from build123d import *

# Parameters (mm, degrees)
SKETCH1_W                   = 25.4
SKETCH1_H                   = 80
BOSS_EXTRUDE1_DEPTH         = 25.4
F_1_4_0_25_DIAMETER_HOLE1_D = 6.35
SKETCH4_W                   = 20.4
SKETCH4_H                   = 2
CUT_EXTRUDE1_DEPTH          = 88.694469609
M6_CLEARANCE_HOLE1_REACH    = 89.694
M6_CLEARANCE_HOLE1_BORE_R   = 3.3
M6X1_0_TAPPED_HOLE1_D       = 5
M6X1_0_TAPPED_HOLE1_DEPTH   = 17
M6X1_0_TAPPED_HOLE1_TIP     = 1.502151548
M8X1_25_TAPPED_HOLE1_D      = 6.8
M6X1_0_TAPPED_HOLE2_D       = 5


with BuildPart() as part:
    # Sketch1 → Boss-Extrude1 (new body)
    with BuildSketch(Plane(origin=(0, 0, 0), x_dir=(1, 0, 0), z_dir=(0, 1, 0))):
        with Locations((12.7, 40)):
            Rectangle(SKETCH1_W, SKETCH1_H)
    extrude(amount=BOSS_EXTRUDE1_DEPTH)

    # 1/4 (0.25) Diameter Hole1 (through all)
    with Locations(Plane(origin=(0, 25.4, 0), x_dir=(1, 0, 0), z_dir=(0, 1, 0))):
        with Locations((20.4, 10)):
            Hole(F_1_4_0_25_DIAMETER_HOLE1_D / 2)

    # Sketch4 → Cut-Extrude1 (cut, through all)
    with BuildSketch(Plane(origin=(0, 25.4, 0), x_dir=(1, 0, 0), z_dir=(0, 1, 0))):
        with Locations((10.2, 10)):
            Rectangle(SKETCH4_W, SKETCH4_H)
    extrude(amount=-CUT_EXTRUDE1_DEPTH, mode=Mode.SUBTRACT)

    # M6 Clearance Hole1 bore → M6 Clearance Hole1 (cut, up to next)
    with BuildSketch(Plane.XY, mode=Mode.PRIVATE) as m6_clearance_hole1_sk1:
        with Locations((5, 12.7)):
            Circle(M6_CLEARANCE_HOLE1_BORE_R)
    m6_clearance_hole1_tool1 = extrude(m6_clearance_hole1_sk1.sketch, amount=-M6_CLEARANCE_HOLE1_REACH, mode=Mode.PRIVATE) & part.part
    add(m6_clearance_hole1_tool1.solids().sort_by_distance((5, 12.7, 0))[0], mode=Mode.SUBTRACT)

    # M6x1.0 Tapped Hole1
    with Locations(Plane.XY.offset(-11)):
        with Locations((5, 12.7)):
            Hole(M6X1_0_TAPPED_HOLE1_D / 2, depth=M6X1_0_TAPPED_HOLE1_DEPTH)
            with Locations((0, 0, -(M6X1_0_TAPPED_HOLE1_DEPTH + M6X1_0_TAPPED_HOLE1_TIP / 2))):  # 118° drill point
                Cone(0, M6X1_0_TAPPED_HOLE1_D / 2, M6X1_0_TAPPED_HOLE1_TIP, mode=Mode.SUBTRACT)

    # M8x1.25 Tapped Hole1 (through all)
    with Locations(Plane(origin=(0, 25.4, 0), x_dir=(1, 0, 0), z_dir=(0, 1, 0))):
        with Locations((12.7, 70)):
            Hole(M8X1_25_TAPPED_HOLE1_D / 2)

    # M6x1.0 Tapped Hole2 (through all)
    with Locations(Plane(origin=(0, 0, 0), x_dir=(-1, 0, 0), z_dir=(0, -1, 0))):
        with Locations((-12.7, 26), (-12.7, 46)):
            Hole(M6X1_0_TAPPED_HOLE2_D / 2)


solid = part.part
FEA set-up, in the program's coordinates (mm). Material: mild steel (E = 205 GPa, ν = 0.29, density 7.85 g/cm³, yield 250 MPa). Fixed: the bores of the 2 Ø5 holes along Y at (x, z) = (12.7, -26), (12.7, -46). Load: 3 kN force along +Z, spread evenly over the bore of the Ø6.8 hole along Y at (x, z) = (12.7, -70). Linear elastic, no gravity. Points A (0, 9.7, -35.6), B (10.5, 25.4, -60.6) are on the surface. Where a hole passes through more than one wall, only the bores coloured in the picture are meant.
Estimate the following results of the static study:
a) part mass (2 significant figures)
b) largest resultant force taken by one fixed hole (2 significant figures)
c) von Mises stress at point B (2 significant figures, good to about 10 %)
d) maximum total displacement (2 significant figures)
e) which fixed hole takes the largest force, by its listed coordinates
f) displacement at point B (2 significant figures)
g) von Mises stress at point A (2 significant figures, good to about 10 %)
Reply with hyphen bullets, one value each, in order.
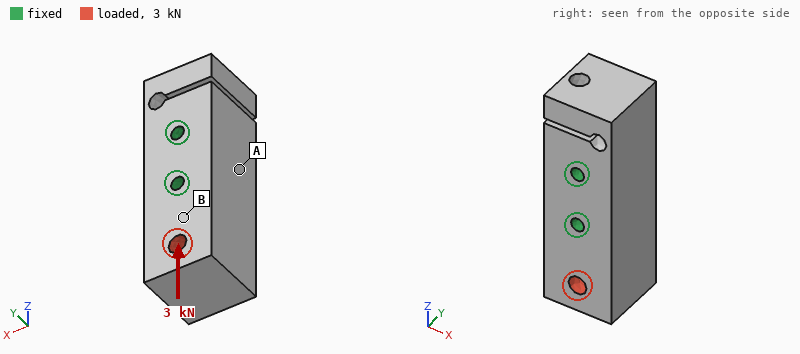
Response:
- 370 g
- 2.4 kN
- 6.5 MPa
- 0.97 µm
- (12.7, -46)
- 0.44 µm
- 1.4 MPa
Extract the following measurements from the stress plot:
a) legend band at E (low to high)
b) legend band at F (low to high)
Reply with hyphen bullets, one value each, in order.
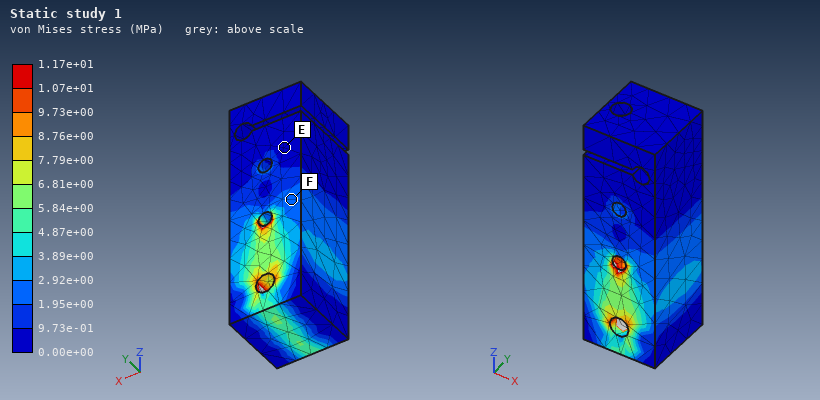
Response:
- 0.00e+00 to 9.73e-01 MPa
- 1.95e+00 to 2.92e+00 MPa
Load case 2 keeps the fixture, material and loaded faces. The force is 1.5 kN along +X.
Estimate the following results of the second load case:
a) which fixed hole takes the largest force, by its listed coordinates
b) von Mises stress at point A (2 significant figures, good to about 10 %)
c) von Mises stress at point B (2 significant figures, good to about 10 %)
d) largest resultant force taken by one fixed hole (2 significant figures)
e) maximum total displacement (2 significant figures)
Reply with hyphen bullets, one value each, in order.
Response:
- (12.7, -46)
- 4.9 MPa
- 6.6 MPa
- 2.7 kN
- 4.7 µm
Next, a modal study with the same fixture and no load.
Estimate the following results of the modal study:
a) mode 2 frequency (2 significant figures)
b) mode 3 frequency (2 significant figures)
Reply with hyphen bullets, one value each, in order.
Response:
- 4000 Hz
- 8500 Hz
